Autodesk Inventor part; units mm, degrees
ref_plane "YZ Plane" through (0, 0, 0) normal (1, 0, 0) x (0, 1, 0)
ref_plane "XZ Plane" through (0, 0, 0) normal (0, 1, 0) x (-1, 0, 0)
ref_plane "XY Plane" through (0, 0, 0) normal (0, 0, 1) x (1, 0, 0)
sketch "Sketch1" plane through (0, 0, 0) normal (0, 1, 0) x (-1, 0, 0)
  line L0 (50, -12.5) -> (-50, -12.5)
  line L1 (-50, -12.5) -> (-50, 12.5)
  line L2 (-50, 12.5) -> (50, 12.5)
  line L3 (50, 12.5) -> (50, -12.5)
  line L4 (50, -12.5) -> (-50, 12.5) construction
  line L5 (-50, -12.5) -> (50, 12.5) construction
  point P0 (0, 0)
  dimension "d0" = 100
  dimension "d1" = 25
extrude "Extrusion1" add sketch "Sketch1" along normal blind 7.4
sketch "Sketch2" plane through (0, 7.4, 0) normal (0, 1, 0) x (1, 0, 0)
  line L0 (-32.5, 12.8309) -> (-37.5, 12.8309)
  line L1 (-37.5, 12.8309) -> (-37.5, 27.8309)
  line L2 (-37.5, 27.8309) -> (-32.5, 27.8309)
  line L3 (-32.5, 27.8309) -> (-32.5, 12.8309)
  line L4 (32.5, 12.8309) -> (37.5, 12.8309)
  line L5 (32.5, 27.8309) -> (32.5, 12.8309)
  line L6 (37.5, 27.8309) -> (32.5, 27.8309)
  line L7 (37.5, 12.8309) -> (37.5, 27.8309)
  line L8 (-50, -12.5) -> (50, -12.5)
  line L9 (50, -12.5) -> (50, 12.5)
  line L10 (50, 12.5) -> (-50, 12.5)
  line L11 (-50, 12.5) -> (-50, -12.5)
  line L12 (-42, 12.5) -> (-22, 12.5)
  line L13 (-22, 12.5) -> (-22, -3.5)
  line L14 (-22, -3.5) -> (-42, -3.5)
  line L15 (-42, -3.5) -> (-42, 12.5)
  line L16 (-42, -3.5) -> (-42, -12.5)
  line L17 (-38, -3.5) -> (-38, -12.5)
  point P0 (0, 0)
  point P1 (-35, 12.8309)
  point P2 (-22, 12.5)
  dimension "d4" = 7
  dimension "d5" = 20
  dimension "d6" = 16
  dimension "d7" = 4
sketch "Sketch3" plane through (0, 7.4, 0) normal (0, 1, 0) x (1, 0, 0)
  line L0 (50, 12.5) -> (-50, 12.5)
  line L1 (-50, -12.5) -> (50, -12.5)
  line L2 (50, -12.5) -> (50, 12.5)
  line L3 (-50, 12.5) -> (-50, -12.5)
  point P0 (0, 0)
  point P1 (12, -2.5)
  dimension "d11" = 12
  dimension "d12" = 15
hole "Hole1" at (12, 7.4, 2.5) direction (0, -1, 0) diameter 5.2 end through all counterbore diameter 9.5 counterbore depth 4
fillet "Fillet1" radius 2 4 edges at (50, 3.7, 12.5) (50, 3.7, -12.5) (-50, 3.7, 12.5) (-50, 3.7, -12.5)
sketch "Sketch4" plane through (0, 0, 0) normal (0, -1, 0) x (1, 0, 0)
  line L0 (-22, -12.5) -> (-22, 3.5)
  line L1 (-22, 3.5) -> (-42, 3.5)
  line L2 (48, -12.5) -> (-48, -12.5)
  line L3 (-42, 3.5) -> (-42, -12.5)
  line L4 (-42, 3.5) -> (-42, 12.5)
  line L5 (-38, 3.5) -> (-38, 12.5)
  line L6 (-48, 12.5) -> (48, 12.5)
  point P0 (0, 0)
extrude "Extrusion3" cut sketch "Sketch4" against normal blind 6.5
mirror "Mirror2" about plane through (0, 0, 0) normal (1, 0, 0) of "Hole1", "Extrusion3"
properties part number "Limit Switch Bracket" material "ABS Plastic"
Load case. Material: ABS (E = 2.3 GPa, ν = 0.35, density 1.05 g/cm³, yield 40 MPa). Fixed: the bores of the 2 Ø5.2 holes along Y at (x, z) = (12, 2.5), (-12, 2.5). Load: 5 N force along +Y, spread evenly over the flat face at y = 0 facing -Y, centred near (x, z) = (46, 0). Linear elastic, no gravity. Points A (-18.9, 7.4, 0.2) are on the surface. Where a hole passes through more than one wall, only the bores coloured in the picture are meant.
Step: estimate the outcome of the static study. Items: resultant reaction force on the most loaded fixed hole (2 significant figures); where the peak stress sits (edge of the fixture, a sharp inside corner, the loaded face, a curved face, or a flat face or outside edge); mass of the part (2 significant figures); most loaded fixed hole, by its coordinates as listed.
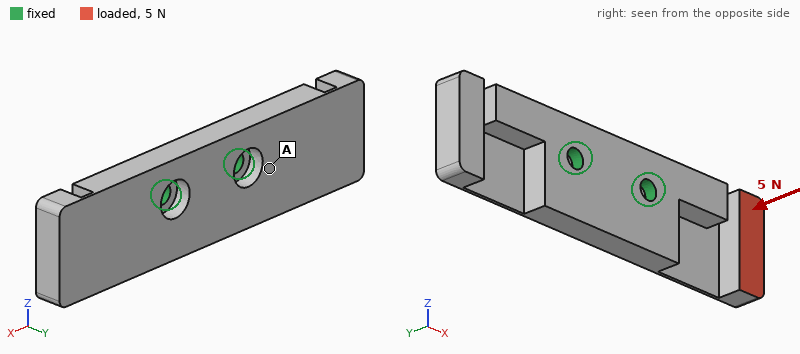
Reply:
13 N
a flat face or outside edge
14 g
(12, 2.5)
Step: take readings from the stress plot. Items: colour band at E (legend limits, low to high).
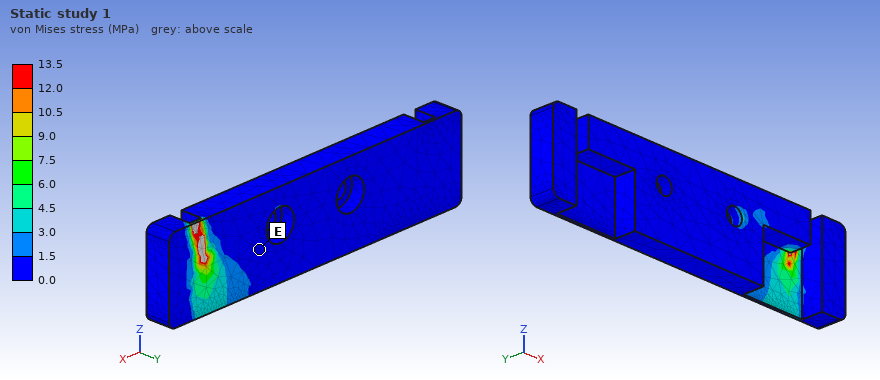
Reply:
0.0 to 1.5 MPa
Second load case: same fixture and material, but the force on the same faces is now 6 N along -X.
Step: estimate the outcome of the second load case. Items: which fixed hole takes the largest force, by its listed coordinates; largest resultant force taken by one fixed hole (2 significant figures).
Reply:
(12, 2.5)
5.6 N
